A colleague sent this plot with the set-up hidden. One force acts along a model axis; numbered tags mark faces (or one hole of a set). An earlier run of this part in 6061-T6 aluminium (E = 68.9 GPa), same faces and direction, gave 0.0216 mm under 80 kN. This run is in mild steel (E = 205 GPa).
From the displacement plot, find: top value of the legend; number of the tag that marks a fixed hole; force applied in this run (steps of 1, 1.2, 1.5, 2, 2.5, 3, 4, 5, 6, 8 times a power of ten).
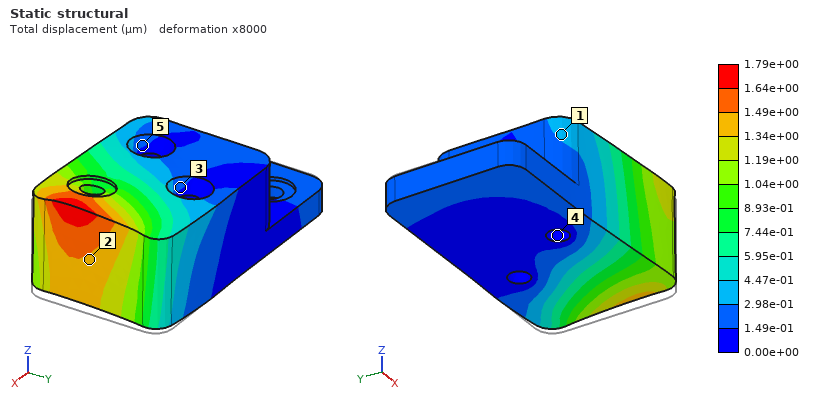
1.79e+00 µm
4
20 kN
